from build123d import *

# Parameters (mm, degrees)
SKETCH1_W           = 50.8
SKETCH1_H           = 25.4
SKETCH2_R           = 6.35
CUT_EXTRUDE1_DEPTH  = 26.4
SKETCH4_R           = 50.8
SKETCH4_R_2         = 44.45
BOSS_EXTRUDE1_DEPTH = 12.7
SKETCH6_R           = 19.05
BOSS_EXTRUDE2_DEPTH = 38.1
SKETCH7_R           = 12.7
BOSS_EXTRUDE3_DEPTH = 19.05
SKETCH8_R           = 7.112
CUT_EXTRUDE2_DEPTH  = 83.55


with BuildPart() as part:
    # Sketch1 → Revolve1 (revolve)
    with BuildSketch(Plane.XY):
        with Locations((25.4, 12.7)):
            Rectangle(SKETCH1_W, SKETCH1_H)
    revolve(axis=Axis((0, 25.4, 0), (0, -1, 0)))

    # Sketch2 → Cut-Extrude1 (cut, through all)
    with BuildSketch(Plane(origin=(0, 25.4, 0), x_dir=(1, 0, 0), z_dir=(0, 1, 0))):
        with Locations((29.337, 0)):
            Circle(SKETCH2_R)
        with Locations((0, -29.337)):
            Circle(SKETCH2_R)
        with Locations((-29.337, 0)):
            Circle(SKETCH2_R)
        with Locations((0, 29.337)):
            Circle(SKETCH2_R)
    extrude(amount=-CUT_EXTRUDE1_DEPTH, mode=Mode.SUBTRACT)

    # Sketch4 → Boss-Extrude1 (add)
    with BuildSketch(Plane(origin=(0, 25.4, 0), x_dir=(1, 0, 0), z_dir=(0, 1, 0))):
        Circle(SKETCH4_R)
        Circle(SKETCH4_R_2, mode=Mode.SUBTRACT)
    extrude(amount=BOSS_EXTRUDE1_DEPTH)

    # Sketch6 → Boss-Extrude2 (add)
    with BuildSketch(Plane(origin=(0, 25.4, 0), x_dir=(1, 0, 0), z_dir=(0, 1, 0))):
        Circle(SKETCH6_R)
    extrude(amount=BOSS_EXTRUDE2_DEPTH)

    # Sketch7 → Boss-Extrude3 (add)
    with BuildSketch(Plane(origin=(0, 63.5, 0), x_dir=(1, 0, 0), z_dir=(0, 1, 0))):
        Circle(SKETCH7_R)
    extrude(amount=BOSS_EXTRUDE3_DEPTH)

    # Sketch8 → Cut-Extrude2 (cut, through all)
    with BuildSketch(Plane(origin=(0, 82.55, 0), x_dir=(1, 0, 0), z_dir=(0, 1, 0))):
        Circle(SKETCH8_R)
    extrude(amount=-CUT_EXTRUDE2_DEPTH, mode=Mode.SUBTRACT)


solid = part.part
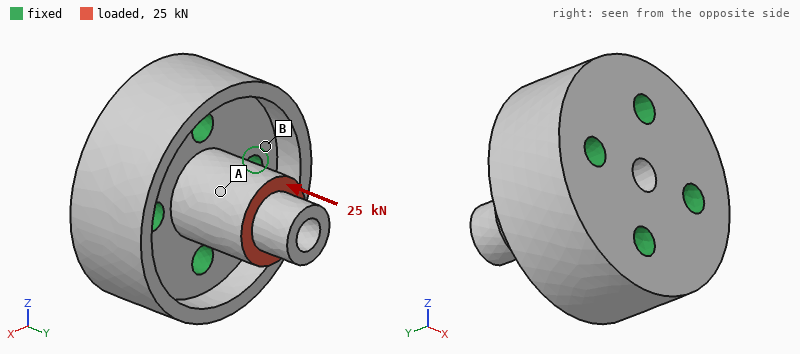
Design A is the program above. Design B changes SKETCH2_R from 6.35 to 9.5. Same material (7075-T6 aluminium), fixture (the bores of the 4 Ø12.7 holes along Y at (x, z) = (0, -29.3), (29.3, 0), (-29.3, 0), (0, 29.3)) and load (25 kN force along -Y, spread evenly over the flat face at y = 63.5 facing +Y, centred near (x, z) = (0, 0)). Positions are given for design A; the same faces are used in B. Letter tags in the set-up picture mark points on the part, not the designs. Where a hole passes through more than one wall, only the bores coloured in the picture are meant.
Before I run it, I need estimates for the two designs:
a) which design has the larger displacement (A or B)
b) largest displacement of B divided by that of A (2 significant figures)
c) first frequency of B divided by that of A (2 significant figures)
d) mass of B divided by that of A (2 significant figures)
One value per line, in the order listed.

A
0.92
1.1
0.94
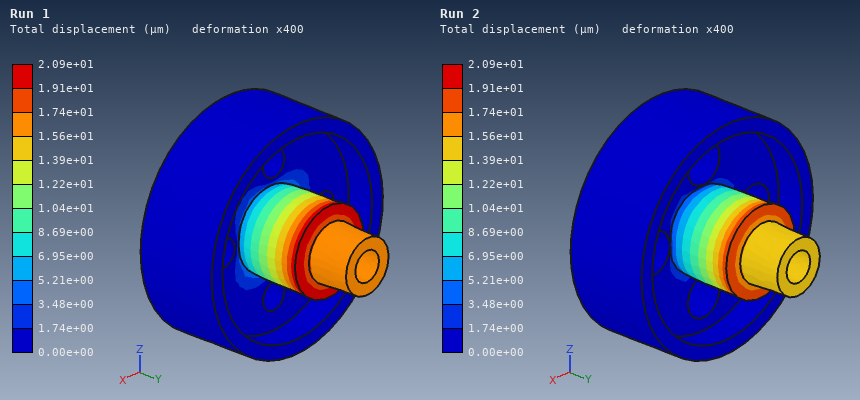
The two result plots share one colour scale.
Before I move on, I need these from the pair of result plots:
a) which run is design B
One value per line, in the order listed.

Run 2
